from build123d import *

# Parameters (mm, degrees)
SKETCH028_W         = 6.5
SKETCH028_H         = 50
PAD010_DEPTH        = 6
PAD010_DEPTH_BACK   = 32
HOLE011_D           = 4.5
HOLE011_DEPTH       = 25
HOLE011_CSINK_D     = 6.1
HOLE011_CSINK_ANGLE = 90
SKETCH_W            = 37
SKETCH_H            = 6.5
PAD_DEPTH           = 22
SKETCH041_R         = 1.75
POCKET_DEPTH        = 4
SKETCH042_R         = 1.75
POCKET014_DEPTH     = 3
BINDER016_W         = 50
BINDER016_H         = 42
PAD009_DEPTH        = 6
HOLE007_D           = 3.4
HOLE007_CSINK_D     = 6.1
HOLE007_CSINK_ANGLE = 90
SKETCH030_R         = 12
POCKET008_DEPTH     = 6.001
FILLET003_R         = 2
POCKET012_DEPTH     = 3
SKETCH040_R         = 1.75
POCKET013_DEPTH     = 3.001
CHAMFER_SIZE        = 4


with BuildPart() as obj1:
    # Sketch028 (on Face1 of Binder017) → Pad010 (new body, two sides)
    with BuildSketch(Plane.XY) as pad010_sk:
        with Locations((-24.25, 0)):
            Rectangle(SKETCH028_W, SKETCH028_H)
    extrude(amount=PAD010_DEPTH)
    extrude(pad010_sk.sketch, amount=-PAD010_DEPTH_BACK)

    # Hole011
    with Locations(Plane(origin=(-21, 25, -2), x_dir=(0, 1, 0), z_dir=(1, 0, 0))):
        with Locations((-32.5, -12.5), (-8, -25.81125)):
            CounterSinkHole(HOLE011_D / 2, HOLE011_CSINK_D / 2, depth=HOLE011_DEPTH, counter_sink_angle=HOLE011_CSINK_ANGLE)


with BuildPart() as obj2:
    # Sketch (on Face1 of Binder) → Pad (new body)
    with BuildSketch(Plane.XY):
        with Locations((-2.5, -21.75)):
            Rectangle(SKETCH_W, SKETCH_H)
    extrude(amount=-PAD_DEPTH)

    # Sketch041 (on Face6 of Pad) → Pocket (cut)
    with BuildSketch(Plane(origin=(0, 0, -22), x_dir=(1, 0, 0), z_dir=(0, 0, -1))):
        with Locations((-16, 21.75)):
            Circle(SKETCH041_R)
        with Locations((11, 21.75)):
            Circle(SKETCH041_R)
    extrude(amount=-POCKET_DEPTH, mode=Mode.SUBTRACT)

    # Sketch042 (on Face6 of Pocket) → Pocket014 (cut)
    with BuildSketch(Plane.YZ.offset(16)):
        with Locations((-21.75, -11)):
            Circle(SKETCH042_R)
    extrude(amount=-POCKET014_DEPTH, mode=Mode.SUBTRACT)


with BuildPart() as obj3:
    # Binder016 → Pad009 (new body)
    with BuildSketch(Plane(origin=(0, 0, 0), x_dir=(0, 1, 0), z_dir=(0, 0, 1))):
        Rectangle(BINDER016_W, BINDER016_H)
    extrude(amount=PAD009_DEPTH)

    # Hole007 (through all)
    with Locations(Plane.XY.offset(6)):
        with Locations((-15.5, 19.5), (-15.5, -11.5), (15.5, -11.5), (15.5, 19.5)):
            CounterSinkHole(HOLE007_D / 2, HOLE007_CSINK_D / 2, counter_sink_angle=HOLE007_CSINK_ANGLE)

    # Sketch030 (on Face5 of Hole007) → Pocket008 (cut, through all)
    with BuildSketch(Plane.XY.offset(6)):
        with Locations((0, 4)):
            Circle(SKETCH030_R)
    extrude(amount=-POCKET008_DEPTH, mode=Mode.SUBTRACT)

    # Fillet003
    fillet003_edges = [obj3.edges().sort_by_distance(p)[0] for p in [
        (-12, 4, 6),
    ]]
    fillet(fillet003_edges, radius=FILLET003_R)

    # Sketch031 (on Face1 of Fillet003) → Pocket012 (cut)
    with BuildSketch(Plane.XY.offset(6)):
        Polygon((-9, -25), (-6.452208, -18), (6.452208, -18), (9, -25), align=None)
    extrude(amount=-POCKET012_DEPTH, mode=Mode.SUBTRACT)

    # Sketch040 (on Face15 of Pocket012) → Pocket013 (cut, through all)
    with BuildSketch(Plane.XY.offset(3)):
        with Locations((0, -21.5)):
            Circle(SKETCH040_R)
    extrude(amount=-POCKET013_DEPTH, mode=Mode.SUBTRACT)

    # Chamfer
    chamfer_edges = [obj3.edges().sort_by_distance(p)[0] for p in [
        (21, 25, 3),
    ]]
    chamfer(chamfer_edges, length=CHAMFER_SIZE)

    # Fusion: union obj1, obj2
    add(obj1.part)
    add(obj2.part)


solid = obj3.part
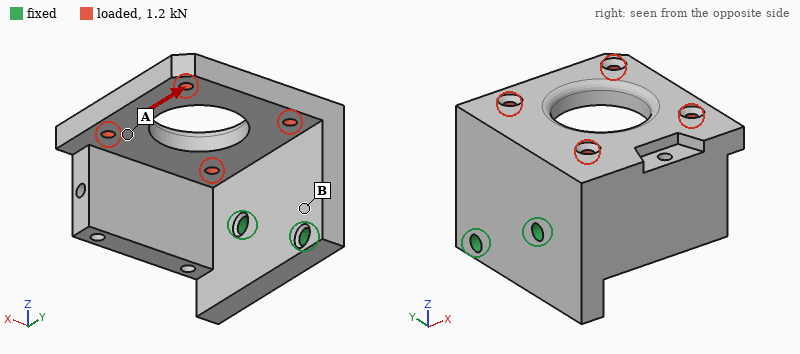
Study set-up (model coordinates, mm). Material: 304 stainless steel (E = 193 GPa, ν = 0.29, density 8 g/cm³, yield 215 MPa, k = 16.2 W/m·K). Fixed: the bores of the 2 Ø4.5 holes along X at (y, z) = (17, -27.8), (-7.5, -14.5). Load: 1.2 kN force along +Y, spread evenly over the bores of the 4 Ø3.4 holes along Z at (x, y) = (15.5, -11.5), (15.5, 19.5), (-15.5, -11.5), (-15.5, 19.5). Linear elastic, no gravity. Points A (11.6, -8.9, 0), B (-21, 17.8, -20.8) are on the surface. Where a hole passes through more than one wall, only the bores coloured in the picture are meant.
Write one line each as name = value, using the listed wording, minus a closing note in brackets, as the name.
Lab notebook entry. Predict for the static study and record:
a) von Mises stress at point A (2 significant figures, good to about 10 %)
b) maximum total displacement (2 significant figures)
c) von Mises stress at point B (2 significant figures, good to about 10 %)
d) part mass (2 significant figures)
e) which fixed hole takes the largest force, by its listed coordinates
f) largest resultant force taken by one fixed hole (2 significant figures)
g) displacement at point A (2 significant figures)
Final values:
von Mises stress at point A = 19 MPa
maximum total displacement = 67 µm
von Mises stress at point B = 41 MPa
part mass = 210 g
which fixed hole takes the largest force, by its listed coordinates = (-7.5, -14.5)
largest resultant force taken by one fixed hole = 1.5 kN
displacement at point A = 47 µm
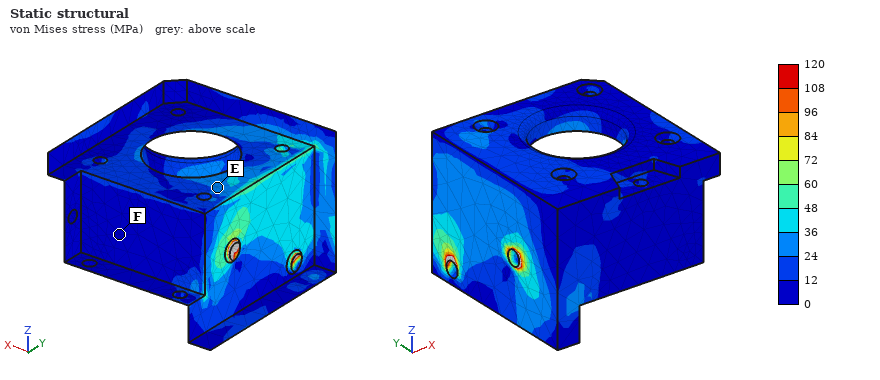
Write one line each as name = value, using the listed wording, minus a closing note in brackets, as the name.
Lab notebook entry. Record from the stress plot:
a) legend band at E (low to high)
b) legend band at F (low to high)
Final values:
legend band at E = 24 to 36 MPa
legend band at F = 0 to 12 MPa
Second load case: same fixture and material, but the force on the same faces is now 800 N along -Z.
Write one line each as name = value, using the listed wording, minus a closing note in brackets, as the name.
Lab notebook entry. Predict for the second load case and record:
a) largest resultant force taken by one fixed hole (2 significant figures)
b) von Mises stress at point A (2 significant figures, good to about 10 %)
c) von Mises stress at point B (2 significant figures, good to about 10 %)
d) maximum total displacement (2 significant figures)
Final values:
largest resultant force taken by one fixed hole = 460 N
von Mises stress at point A = 23 MPa
von Mises stress at point B = 24 MPa
maximum total displacement = 0.11 mm
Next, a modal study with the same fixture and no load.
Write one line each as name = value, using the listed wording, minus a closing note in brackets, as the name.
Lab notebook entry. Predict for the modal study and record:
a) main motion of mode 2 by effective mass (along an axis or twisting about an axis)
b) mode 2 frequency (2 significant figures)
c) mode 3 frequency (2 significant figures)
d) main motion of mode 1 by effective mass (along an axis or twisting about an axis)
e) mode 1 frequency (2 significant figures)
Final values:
main motion of mode 2 by effective mass = along Y
mode 2 frequency = 2300 Hz
mode 3 frequency = 4100 Hz
main motion of mode 1 by effective mass = along Z
mode 1 frequency = 1900 Hz
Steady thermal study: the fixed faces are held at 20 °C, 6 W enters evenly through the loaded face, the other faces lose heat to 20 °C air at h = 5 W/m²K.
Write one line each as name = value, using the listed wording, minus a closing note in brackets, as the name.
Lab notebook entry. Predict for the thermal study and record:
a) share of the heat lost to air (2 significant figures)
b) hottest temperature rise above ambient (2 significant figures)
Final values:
share of the heat lost to air = 20 %
hottest temperature rise above ambient = 59 K
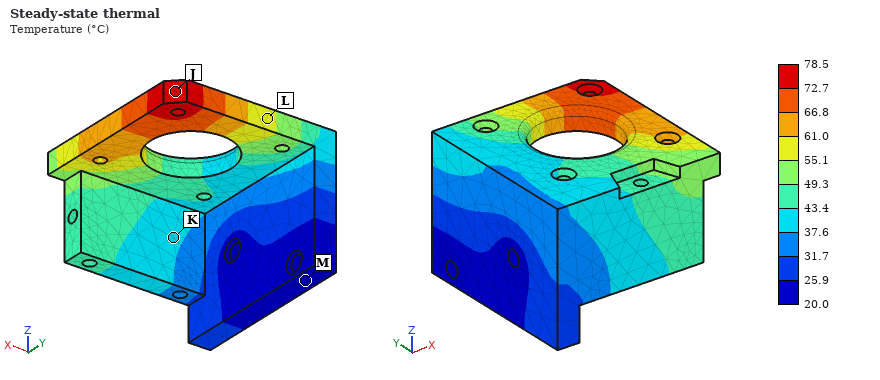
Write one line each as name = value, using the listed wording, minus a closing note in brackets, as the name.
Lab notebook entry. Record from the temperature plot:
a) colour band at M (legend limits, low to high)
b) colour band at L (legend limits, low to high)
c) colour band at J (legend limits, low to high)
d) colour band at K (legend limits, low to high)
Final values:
colour band at M = 20.0 to 25.9 °C
colour band at L = 55.1 to 61.0 °C
colour band at J = 72.7 to 78.5 °C
colour band at K = 37.6 to 43.4 °C
